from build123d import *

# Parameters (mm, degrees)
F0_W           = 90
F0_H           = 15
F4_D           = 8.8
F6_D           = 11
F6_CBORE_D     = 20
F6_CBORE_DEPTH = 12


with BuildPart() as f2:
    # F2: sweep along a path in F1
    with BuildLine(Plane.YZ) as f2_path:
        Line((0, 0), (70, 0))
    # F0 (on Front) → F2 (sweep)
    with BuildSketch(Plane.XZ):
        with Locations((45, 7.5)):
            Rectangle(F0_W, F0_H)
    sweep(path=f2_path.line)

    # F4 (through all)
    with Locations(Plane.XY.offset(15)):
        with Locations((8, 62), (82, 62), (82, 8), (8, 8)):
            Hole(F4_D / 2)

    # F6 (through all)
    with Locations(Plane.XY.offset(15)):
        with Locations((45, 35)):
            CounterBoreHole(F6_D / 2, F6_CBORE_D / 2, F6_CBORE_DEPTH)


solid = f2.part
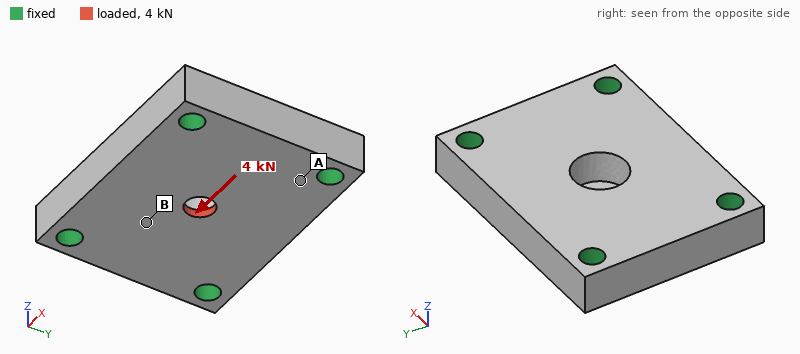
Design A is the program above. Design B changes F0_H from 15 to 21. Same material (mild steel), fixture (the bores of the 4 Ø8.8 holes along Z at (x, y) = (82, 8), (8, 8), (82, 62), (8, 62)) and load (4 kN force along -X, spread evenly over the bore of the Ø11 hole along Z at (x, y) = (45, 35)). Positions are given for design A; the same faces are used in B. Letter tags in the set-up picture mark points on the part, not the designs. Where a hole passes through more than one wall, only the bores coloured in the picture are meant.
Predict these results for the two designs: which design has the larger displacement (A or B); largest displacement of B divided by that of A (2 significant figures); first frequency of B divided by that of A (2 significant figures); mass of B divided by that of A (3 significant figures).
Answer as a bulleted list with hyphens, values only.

- A
- 0.59
- 1.2
- 1.40
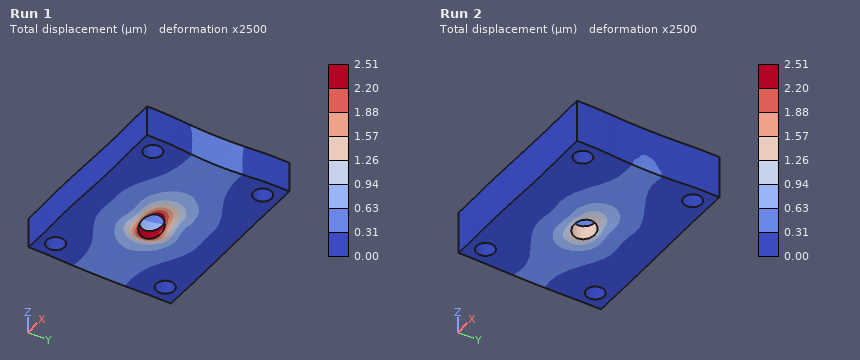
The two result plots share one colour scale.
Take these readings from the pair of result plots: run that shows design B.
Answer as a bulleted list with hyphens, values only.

- Run 2
